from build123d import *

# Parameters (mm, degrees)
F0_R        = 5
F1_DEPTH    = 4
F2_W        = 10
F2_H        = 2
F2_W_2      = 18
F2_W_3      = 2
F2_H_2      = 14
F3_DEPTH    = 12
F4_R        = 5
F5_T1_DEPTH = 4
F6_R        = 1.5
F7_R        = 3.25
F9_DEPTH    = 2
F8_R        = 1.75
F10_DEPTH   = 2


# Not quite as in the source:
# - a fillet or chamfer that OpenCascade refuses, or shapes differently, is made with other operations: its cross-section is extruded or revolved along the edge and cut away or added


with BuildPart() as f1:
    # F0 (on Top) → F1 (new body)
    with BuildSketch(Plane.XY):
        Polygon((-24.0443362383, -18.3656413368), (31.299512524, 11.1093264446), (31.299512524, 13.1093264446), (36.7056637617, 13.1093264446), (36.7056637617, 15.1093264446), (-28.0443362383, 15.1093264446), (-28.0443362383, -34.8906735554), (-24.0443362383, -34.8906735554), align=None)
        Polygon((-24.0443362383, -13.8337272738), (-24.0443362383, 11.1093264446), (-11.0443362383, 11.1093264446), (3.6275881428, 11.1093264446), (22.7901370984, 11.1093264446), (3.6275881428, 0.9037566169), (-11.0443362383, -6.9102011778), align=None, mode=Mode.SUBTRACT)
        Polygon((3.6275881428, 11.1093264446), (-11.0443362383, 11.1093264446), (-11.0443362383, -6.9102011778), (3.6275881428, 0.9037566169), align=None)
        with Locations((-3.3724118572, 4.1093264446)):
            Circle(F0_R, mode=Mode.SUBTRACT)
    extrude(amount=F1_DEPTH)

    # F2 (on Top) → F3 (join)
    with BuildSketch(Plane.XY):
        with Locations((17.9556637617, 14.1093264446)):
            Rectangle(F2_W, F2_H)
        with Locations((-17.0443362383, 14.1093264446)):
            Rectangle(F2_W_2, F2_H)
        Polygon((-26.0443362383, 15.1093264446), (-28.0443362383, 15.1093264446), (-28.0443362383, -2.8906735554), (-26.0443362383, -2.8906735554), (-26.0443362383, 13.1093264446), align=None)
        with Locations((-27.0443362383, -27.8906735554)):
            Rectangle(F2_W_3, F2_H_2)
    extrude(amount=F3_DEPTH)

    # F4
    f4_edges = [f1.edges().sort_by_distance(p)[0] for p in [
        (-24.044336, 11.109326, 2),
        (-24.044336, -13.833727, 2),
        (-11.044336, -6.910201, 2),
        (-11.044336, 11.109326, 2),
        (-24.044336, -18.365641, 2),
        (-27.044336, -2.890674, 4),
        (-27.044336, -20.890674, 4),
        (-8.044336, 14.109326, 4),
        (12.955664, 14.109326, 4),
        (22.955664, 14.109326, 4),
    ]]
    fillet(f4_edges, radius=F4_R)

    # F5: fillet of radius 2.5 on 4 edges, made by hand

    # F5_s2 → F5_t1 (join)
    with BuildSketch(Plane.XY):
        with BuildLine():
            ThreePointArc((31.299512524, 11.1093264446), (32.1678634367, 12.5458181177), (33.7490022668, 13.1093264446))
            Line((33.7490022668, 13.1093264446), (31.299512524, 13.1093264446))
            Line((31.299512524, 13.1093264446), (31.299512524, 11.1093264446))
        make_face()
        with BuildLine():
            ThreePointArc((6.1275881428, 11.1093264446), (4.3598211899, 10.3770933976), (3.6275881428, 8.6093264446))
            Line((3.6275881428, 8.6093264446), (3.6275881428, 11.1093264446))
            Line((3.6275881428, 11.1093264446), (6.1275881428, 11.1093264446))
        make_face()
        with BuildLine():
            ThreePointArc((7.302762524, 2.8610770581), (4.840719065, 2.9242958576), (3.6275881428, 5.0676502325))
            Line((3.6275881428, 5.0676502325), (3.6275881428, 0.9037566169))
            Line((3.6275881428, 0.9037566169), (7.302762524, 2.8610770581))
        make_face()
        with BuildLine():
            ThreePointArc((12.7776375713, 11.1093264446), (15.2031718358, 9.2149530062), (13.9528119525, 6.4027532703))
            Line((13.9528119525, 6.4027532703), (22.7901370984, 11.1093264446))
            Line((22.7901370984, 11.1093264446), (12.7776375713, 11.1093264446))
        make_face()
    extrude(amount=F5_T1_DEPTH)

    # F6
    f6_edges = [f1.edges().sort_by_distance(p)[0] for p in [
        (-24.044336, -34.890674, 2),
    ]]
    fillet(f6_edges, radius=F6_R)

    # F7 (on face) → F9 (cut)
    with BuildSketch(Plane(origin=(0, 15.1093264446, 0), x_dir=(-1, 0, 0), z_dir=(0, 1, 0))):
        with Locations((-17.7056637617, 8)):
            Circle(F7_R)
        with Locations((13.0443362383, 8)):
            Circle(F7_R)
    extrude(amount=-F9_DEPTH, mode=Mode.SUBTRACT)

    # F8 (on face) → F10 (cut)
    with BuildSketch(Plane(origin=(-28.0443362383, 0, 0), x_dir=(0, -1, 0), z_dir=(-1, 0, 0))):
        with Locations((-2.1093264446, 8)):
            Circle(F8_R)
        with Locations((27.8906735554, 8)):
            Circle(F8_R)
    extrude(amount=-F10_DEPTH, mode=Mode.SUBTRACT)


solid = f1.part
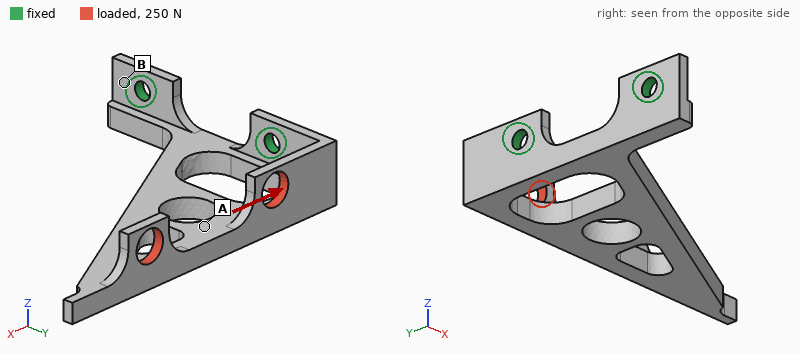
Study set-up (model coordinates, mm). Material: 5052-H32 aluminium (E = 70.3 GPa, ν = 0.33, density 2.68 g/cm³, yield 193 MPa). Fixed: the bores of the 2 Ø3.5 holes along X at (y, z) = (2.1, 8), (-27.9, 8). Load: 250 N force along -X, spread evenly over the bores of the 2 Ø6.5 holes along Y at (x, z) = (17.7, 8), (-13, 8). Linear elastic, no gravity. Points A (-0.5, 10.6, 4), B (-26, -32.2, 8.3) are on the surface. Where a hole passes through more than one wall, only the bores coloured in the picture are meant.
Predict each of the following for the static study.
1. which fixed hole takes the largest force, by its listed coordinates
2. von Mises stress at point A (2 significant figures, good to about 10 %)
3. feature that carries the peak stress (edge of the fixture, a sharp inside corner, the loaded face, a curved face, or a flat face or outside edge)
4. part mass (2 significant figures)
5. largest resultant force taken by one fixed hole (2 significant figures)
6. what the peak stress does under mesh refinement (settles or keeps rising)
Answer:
(2.1, 8)
26 MPa
edge of the fixture
11 g
320 N
keeps rising
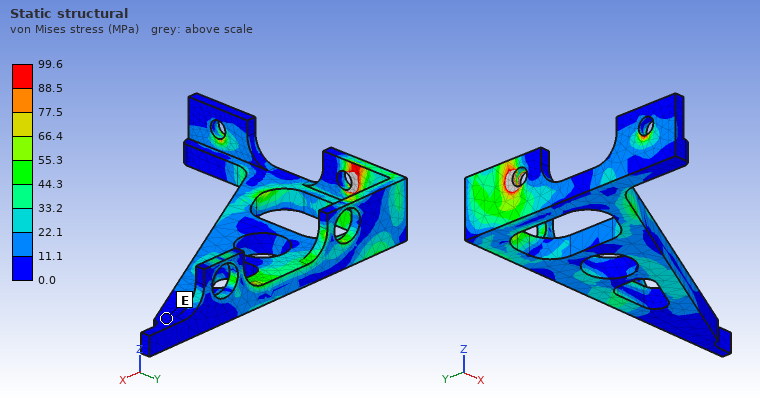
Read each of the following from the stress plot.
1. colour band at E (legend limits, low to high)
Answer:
0.0 to 11.1 MPa
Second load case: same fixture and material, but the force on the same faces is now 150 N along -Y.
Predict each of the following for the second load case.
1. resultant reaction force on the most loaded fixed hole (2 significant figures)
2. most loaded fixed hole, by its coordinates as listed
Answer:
180 N
(-27.9, 8)
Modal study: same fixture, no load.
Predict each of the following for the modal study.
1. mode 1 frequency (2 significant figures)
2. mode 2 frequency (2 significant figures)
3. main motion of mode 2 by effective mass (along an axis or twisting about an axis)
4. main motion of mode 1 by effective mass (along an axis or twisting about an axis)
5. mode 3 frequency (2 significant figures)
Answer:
740 Hz
2500 Hz
along Y
along Z
3900 Hz
